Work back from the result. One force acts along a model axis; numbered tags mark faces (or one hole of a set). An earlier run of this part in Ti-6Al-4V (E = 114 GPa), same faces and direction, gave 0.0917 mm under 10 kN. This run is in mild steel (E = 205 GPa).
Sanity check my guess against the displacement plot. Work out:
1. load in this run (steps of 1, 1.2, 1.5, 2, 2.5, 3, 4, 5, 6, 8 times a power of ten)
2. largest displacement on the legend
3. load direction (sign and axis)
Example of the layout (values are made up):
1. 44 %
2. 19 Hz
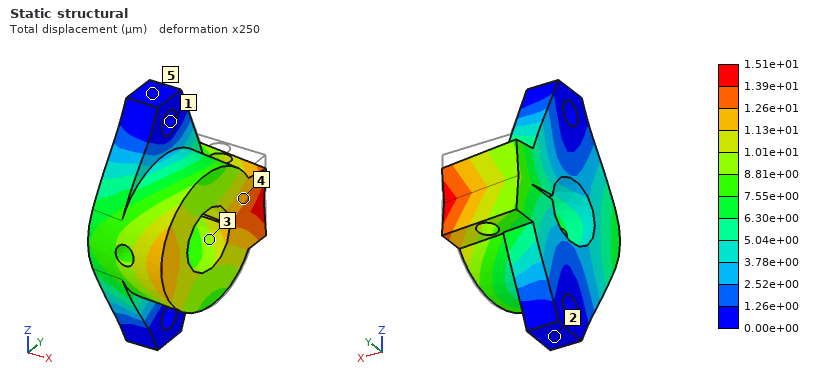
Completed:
1. 3 kN
2. 1.51e+01 µm
3. -Y
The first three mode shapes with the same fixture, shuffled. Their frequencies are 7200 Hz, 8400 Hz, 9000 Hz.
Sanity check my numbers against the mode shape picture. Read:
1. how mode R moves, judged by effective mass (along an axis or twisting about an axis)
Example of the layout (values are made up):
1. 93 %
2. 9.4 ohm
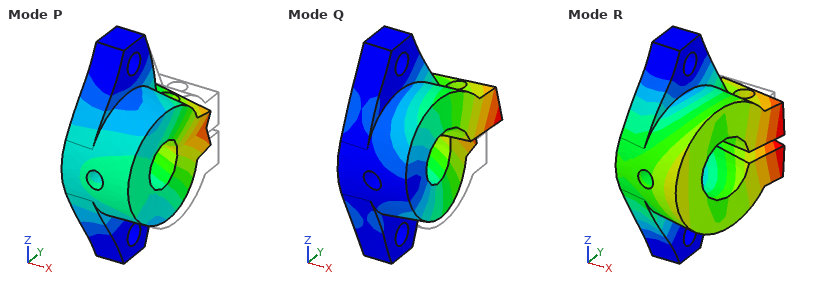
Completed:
1. along Y
